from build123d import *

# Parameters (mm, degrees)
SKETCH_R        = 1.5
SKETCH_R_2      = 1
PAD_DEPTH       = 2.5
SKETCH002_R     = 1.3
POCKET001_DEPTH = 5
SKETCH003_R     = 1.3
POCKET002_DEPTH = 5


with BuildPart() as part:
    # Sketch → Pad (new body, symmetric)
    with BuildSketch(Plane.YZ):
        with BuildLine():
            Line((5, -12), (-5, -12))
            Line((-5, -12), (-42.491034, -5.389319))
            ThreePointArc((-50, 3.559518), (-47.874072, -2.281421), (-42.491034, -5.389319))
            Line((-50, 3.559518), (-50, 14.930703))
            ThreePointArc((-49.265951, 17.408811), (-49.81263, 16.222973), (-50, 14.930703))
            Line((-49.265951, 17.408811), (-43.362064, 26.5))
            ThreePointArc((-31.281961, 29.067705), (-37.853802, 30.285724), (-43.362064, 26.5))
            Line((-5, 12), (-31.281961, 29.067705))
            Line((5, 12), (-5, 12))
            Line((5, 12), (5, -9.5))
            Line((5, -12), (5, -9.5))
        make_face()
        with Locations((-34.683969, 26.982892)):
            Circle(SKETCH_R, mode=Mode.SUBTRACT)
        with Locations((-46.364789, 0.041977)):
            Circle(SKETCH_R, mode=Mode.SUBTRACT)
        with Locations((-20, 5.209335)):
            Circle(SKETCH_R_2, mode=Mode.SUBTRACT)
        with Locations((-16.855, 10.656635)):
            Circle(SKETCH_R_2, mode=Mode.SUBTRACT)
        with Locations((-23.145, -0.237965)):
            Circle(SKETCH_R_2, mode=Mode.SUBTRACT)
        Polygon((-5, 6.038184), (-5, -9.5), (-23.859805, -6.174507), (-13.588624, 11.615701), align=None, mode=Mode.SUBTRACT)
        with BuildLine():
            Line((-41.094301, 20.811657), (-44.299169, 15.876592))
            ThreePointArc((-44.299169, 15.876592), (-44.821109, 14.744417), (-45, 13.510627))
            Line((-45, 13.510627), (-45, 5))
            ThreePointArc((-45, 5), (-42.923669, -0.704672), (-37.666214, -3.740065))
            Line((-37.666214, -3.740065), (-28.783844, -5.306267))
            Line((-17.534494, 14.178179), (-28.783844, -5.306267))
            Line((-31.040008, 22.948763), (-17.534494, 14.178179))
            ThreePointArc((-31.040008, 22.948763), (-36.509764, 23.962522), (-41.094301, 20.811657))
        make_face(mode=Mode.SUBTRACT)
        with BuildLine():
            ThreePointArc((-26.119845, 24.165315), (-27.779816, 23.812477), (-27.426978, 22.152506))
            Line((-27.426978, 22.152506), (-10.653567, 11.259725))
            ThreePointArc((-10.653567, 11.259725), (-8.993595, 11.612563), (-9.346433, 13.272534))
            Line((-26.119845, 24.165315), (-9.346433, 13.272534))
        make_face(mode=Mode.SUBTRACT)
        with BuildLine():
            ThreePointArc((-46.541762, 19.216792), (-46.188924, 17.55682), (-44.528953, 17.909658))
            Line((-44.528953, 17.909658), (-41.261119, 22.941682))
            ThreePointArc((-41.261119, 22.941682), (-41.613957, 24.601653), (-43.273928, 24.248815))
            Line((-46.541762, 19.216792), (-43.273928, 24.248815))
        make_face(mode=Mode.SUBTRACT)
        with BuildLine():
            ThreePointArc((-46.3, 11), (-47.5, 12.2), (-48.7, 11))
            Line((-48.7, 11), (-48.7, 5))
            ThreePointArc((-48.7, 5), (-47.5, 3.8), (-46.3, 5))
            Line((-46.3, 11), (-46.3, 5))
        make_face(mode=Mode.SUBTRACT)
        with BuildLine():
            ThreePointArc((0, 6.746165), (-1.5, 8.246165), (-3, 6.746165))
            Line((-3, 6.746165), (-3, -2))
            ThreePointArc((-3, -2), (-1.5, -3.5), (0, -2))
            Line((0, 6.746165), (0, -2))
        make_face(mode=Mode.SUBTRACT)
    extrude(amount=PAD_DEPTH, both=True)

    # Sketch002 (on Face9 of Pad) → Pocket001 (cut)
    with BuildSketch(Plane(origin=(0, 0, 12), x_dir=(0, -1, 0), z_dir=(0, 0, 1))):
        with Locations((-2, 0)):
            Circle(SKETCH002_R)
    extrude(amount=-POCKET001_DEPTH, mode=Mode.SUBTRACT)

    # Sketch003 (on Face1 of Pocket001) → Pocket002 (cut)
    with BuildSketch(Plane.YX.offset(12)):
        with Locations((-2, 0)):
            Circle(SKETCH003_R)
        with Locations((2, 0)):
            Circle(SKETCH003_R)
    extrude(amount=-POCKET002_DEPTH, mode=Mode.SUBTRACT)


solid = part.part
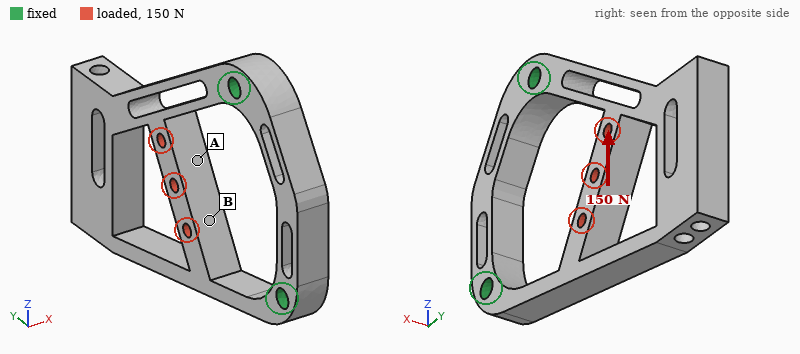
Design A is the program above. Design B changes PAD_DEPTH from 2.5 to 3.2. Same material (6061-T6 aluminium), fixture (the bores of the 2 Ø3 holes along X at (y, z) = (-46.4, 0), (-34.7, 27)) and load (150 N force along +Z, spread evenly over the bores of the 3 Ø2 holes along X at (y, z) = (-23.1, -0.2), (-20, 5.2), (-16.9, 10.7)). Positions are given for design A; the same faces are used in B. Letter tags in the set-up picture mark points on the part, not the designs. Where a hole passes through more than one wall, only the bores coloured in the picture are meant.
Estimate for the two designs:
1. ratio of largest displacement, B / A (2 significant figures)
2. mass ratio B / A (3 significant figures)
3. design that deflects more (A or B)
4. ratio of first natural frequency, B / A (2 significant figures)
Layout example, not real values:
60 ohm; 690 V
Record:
0.77; 1.29; A; 1.3
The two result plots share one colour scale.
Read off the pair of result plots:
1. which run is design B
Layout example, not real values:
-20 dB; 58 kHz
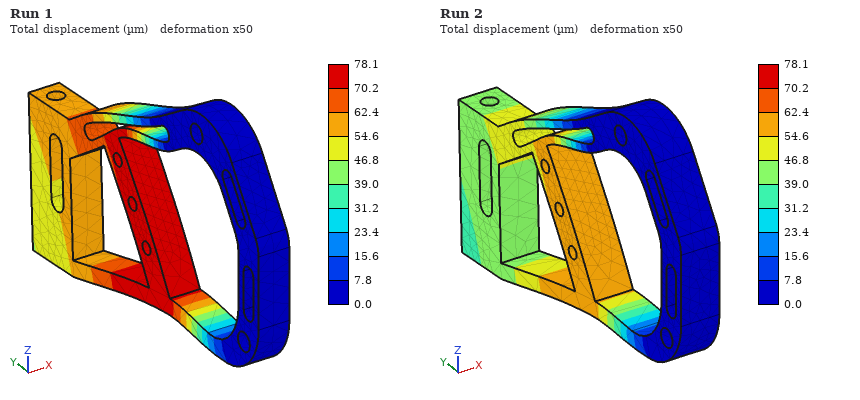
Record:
Run 2
